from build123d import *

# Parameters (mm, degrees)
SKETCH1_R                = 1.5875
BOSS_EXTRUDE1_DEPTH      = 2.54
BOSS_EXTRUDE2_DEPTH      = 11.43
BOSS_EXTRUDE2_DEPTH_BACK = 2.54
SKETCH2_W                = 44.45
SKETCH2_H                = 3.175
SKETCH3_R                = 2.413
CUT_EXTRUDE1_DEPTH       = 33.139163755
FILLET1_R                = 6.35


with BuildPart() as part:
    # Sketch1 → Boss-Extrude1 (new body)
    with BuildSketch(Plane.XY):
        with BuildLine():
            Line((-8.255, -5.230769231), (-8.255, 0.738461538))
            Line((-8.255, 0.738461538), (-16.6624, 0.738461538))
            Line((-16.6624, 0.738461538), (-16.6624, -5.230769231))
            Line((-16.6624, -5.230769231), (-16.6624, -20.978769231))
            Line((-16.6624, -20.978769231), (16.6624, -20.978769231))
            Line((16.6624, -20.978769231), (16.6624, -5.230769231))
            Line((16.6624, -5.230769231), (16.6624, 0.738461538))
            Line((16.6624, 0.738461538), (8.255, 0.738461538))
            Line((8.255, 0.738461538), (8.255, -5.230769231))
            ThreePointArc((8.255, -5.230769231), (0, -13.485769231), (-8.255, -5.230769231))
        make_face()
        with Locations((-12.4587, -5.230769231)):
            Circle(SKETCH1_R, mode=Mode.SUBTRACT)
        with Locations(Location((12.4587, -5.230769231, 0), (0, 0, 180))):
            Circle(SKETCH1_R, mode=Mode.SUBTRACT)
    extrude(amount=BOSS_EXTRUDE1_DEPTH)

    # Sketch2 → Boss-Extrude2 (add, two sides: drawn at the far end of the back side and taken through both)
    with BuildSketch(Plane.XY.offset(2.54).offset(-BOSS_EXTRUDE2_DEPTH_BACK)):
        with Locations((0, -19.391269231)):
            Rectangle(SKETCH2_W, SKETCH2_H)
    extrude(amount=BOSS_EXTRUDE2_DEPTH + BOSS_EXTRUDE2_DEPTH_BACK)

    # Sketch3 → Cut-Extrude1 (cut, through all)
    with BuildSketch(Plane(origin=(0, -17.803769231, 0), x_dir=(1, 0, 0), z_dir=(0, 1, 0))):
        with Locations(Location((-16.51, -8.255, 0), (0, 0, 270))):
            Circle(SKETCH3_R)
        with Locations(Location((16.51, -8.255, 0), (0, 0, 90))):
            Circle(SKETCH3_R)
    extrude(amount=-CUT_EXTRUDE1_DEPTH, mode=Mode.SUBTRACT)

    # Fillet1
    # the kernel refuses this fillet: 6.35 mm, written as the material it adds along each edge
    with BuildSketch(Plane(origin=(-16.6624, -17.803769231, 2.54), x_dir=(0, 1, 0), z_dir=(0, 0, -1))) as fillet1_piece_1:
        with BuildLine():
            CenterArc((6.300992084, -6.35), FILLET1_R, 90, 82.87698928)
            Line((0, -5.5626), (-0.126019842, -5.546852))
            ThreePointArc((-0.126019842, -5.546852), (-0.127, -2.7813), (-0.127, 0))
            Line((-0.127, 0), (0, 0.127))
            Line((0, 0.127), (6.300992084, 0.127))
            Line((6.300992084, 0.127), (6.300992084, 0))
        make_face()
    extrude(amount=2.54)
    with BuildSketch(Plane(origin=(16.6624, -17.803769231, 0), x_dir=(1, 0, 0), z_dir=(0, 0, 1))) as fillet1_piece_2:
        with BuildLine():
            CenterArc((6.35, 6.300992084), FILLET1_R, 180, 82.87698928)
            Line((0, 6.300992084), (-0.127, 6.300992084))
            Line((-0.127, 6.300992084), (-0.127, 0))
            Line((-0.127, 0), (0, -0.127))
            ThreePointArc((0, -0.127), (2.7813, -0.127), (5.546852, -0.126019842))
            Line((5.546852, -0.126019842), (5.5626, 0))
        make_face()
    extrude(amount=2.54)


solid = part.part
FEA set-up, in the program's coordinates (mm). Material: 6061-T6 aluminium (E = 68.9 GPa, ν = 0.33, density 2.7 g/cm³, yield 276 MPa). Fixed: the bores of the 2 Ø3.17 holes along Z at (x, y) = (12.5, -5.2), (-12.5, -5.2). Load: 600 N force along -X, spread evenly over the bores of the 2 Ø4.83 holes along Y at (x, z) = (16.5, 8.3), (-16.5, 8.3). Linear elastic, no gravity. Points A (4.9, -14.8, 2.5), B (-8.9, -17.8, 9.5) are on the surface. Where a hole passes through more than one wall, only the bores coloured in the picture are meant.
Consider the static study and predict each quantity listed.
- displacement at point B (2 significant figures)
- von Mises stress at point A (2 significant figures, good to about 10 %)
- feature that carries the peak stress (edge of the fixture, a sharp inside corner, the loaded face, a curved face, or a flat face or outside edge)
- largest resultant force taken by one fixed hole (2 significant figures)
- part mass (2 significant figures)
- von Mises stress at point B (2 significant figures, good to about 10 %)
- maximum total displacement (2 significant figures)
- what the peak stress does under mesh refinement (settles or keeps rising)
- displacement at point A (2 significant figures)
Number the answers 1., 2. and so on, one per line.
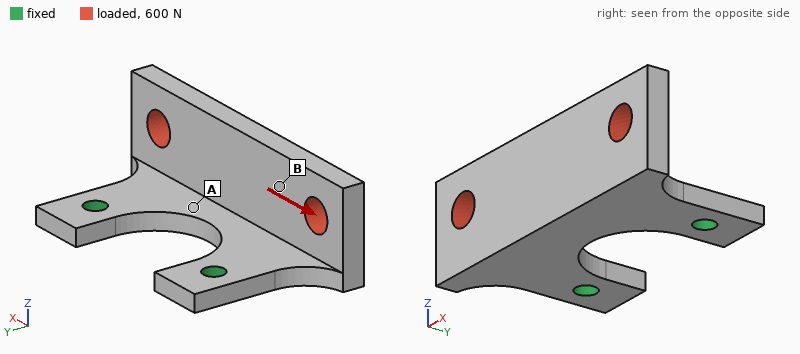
1. 0.053 mm
2. 56 MPa
3. edge of the fixture
4. 420 N
5. 7.8 g
6. 24 MPa
7. 0.11 mm
8. keeps rising
9. 0.016 mm
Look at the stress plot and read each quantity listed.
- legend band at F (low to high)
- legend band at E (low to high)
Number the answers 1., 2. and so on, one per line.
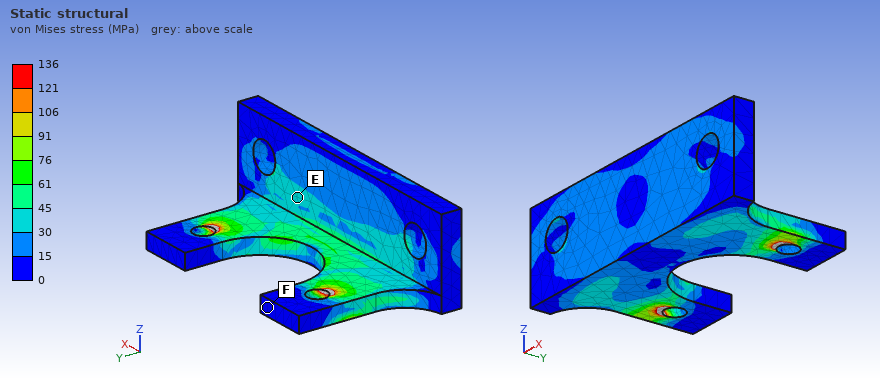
1. 0 to 15 MPa
2. 30 to 45 MPa
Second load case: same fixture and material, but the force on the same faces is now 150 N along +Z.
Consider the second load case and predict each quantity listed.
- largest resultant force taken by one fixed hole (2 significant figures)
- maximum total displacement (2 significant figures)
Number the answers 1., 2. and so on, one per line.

1. 75 N
2. 0.12 mm
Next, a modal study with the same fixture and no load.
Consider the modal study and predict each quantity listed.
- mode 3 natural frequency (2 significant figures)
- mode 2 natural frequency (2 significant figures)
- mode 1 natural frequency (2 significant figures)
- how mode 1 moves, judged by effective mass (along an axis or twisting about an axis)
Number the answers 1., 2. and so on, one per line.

1. 9800 Hz
2. 4900 Hz
3. 2600 Hz
4. along Z
